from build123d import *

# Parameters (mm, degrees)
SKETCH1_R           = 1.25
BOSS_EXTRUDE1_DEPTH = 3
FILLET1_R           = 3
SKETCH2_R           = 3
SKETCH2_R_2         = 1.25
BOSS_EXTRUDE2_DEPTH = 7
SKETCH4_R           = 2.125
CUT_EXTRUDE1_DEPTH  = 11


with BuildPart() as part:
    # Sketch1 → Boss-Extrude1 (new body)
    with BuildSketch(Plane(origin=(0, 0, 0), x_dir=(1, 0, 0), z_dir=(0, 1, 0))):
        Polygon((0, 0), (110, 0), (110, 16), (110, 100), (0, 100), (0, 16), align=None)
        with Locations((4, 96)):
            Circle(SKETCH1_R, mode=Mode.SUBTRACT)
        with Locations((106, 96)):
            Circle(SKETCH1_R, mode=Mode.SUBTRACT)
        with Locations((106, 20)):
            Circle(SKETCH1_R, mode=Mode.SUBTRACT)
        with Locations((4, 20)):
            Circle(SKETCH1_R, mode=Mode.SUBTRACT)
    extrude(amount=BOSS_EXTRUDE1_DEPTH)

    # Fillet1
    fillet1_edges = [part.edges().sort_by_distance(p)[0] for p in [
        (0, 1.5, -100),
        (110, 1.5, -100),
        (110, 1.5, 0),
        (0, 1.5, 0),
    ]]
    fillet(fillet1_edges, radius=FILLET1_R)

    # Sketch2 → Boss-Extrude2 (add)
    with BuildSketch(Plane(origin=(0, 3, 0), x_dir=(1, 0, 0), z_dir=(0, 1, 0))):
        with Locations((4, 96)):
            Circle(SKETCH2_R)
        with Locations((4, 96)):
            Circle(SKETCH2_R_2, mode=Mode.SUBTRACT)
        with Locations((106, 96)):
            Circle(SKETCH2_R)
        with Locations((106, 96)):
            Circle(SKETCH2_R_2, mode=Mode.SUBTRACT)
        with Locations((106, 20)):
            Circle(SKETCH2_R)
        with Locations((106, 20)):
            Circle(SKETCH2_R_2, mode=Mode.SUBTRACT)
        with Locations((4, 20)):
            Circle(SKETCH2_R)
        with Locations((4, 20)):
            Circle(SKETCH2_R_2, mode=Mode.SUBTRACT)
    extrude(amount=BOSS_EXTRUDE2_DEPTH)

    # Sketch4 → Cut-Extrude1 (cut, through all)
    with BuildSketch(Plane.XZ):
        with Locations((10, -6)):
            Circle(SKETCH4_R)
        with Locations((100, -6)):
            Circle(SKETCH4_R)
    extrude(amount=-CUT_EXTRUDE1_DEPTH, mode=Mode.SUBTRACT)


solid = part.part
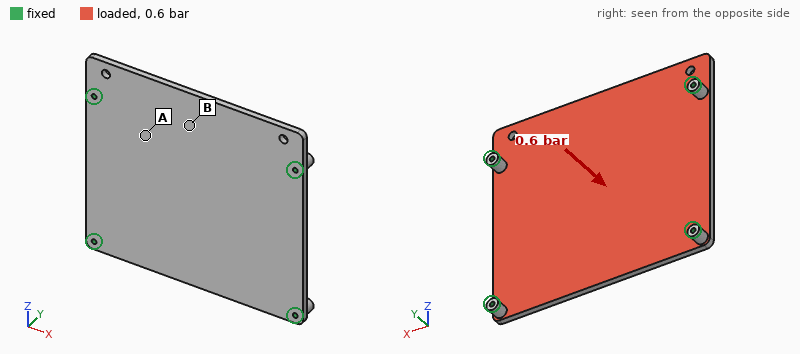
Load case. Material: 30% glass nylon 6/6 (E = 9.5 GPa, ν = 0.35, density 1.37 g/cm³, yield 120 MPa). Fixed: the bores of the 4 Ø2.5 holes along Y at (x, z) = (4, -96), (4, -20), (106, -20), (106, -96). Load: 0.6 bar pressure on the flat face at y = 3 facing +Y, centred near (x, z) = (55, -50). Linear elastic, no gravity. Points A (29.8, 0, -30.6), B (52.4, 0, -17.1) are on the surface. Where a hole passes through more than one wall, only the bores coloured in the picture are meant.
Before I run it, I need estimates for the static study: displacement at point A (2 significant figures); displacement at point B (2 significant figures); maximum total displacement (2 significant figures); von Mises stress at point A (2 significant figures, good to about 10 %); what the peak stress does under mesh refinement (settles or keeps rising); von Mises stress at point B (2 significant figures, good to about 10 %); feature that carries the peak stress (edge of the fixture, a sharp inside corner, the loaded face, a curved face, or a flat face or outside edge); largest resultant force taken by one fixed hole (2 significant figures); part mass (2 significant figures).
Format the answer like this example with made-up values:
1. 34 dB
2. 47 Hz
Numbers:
1. 0.86 mm
2. 1.2 mm
3. 1.4 mm
4. 12 MPa
5. keeps rising
6. 22 MPa
7. edge of the fixture
8. 200 N
9. 46 g
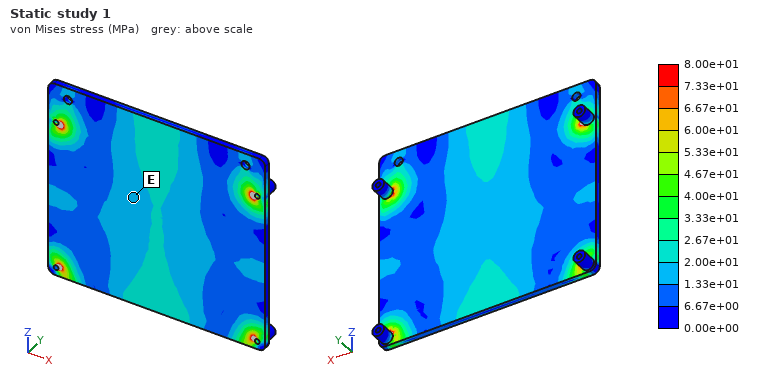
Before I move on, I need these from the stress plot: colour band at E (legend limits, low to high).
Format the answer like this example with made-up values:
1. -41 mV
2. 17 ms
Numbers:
1. 1.33e+01 to 2.00e+01 MPa
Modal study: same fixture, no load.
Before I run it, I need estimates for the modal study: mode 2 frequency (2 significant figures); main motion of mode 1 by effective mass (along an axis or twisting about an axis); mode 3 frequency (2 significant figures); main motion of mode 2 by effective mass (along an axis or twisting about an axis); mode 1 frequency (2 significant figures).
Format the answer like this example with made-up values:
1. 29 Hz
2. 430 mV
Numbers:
1. 830 Hz
2. along Y
3. 1200 Hz
4. twisting about X
5. 600 Hz
